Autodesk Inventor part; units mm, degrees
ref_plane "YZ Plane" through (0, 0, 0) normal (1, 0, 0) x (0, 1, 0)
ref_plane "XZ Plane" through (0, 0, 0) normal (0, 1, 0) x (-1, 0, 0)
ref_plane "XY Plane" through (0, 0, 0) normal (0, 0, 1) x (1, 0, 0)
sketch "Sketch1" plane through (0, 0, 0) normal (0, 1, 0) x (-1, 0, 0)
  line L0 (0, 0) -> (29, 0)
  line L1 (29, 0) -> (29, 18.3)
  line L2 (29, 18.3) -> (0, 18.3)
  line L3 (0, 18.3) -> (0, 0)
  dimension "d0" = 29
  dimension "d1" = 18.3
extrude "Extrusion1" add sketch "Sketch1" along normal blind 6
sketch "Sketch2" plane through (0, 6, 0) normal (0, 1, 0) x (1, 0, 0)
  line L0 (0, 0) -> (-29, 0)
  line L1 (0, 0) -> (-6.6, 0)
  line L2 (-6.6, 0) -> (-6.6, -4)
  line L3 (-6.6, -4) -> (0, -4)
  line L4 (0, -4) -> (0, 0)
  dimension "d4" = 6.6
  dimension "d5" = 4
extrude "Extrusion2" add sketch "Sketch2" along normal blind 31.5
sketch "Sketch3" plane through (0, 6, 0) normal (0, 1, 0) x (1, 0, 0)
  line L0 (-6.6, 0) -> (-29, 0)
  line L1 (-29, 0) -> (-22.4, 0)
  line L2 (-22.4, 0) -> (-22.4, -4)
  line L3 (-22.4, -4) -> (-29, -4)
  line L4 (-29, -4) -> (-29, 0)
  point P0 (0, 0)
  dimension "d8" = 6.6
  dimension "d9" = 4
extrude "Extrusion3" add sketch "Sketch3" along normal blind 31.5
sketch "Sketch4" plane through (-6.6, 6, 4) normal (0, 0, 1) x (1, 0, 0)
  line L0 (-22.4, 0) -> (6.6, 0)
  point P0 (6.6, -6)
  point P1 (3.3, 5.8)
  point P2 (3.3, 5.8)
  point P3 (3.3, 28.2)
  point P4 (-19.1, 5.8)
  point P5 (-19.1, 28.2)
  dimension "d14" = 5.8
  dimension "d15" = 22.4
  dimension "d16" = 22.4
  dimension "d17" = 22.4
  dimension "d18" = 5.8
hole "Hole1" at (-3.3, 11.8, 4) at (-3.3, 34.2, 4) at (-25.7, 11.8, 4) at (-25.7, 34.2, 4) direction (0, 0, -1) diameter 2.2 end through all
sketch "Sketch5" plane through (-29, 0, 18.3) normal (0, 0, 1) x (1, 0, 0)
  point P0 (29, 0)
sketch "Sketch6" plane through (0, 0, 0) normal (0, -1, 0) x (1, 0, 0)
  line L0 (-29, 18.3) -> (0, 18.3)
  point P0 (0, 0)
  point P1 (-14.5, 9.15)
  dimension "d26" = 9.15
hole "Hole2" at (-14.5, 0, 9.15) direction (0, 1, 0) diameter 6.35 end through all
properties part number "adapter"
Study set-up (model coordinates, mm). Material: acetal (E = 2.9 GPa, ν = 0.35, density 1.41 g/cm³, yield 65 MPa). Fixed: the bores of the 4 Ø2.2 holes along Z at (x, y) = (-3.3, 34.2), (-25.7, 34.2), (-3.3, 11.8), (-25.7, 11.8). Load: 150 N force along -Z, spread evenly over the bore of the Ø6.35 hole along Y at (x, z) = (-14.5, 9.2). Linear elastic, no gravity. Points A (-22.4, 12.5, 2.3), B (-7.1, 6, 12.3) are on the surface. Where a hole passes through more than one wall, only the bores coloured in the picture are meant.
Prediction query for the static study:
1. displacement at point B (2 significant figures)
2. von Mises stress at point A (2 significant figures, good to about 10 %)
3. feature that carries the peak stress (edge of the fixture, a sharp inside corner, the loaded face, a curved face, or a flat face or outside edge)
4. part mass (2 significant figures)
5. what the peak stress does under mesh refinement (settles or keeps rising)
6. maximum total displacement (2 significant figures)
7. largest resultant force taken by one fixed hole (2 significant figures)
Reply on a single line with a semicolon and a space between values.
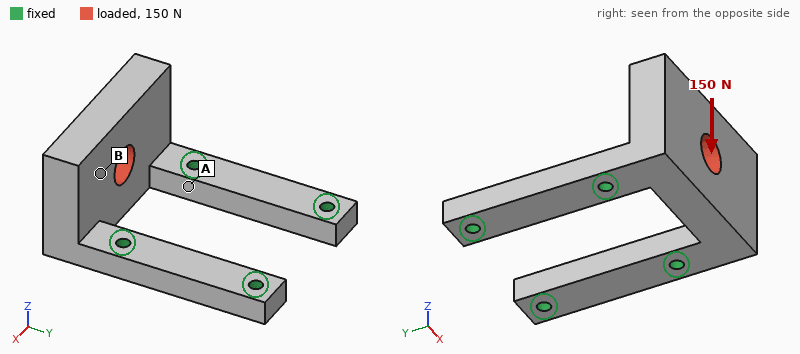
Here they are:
0.29 mm; 7.1 MPa; edge of the fixture; 6.5 g; keeps rising; 0.51 mm; 77 N
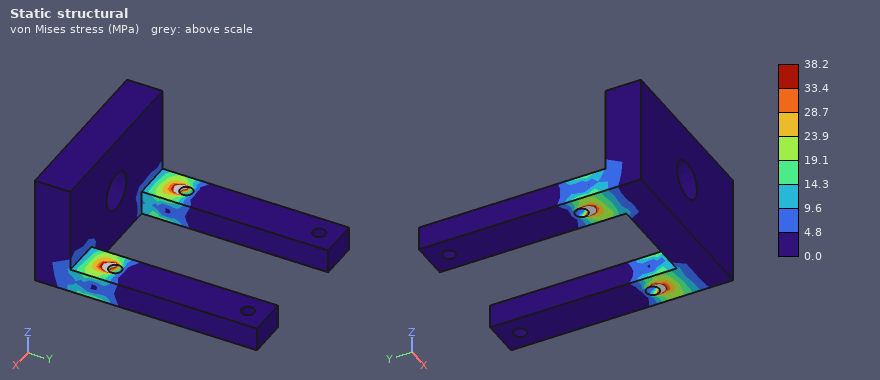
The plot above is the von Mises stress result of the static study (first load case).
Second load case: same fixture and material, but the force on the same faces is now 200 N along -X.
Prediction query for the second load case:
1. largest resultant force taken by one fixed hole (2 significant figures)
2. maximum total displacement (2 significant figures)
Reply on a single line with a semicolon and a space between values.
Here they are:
130 N; 0.15 mm
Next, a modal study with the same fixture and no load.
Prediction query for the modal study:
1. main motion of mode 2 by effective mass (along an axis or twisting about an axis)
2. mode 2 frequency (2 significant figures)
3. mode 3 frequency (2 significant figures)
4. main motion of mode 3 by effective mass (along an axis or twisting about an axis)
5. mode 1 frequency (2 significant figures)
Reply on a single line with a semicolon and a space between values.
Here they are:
along X; 3000 Hz; 4700 Hz; along Z; 1200 Hz
